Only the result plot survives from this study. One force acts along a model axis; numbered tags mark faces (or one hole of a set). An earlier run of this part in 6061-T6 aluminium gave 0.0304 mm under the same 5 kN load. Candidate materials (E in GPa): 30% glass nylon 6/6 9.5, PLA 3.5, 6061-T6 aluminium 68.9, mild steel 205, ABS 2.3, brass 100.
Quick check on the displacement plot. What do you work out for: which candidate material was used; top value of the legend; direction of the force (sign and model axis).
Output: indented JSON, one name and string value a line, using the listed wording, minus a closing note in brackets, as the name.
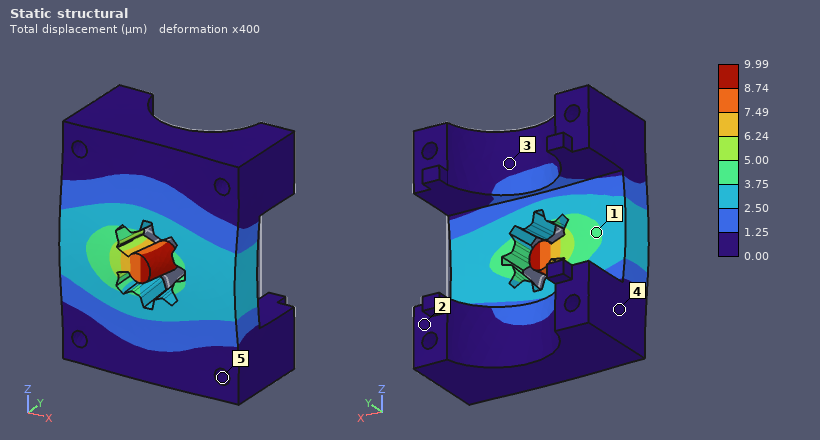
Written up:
{
  "which candidate material was used": "mild steel",
  "top value of the legend": "9.99 µm",
  "direction of the force": "-Y"
}
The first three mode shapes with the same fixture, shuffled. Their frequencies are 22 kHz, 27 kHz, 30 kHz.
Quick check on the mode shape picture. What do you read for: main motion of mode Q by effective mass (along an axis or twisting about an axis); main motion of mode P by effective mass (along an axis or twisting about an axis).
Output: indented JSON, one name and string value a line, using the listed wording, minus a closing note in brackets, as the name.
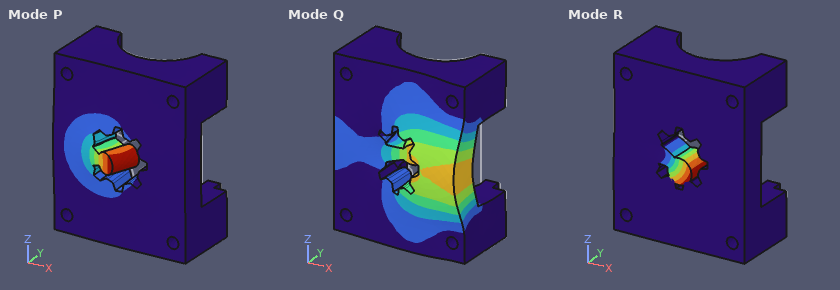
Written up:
{
  "main motion of mode Q by effective mass": "along Y",
  "main motion of mode P by effective mass": "along Y"
}
